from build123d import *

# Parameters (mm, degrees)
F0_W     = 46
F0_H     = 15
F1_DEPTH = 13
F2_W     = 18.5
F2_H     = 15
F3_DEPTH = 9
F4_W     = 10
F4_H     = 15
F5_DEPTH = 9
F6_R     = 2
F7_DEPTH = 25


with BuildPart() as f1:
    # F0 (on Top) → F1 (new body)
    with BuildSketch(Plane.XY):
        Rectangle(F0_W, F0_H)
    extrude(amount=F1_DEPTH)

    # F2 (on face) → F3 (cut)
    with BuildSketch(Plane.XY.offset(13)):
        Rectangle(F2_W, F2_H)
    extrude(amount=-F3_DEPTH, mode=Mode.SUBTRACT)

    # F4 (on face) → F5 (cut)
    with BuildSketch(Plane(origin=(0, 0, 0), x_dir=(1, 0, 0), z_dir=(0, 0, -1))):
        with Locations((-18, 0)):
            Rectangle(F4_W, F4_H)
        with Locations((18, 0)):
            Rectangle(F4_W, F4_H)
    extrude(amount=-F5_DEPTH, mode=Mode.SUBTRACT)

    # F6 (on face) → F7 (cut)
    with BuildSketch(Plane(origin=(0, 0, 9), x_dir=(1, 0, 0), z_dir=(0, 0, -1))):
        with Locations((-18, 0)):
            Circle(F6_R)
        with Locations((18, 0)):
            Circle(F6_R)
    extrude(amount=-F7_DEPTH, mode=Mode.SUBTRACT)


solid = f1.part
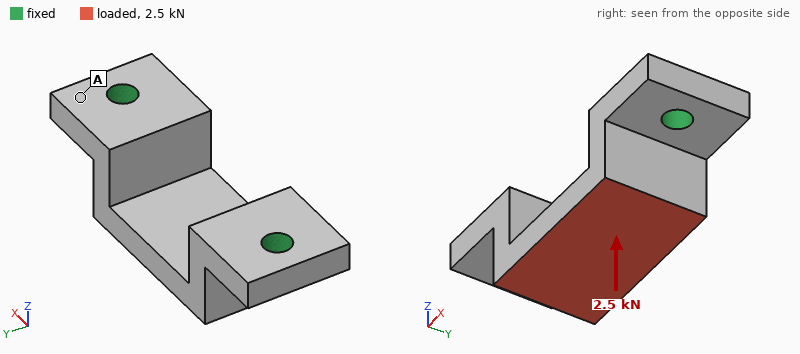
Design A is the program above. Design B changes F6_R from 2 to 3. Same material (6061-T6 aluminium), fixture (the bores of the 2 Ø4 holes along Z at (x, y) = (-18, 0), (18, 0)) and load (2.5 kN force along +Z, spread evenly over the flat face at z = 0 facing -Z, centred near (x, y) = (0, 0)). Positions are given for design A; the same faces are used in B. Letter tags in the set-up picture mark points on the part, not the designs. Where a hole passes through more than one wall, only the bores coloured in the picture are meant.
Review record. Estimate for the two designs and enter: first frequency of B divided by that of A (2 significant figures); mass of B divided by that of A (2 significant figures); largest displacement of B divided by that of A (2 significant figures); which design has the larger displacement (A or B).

1.2
0.97
0.87
A
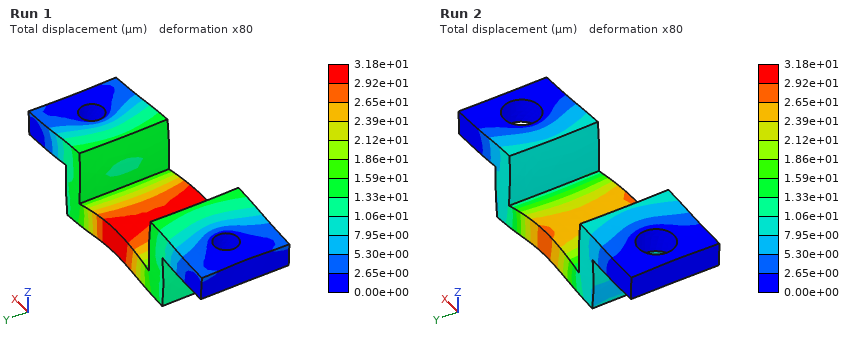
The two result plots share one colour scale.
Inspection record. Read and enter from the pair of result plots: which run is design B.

Run 2
